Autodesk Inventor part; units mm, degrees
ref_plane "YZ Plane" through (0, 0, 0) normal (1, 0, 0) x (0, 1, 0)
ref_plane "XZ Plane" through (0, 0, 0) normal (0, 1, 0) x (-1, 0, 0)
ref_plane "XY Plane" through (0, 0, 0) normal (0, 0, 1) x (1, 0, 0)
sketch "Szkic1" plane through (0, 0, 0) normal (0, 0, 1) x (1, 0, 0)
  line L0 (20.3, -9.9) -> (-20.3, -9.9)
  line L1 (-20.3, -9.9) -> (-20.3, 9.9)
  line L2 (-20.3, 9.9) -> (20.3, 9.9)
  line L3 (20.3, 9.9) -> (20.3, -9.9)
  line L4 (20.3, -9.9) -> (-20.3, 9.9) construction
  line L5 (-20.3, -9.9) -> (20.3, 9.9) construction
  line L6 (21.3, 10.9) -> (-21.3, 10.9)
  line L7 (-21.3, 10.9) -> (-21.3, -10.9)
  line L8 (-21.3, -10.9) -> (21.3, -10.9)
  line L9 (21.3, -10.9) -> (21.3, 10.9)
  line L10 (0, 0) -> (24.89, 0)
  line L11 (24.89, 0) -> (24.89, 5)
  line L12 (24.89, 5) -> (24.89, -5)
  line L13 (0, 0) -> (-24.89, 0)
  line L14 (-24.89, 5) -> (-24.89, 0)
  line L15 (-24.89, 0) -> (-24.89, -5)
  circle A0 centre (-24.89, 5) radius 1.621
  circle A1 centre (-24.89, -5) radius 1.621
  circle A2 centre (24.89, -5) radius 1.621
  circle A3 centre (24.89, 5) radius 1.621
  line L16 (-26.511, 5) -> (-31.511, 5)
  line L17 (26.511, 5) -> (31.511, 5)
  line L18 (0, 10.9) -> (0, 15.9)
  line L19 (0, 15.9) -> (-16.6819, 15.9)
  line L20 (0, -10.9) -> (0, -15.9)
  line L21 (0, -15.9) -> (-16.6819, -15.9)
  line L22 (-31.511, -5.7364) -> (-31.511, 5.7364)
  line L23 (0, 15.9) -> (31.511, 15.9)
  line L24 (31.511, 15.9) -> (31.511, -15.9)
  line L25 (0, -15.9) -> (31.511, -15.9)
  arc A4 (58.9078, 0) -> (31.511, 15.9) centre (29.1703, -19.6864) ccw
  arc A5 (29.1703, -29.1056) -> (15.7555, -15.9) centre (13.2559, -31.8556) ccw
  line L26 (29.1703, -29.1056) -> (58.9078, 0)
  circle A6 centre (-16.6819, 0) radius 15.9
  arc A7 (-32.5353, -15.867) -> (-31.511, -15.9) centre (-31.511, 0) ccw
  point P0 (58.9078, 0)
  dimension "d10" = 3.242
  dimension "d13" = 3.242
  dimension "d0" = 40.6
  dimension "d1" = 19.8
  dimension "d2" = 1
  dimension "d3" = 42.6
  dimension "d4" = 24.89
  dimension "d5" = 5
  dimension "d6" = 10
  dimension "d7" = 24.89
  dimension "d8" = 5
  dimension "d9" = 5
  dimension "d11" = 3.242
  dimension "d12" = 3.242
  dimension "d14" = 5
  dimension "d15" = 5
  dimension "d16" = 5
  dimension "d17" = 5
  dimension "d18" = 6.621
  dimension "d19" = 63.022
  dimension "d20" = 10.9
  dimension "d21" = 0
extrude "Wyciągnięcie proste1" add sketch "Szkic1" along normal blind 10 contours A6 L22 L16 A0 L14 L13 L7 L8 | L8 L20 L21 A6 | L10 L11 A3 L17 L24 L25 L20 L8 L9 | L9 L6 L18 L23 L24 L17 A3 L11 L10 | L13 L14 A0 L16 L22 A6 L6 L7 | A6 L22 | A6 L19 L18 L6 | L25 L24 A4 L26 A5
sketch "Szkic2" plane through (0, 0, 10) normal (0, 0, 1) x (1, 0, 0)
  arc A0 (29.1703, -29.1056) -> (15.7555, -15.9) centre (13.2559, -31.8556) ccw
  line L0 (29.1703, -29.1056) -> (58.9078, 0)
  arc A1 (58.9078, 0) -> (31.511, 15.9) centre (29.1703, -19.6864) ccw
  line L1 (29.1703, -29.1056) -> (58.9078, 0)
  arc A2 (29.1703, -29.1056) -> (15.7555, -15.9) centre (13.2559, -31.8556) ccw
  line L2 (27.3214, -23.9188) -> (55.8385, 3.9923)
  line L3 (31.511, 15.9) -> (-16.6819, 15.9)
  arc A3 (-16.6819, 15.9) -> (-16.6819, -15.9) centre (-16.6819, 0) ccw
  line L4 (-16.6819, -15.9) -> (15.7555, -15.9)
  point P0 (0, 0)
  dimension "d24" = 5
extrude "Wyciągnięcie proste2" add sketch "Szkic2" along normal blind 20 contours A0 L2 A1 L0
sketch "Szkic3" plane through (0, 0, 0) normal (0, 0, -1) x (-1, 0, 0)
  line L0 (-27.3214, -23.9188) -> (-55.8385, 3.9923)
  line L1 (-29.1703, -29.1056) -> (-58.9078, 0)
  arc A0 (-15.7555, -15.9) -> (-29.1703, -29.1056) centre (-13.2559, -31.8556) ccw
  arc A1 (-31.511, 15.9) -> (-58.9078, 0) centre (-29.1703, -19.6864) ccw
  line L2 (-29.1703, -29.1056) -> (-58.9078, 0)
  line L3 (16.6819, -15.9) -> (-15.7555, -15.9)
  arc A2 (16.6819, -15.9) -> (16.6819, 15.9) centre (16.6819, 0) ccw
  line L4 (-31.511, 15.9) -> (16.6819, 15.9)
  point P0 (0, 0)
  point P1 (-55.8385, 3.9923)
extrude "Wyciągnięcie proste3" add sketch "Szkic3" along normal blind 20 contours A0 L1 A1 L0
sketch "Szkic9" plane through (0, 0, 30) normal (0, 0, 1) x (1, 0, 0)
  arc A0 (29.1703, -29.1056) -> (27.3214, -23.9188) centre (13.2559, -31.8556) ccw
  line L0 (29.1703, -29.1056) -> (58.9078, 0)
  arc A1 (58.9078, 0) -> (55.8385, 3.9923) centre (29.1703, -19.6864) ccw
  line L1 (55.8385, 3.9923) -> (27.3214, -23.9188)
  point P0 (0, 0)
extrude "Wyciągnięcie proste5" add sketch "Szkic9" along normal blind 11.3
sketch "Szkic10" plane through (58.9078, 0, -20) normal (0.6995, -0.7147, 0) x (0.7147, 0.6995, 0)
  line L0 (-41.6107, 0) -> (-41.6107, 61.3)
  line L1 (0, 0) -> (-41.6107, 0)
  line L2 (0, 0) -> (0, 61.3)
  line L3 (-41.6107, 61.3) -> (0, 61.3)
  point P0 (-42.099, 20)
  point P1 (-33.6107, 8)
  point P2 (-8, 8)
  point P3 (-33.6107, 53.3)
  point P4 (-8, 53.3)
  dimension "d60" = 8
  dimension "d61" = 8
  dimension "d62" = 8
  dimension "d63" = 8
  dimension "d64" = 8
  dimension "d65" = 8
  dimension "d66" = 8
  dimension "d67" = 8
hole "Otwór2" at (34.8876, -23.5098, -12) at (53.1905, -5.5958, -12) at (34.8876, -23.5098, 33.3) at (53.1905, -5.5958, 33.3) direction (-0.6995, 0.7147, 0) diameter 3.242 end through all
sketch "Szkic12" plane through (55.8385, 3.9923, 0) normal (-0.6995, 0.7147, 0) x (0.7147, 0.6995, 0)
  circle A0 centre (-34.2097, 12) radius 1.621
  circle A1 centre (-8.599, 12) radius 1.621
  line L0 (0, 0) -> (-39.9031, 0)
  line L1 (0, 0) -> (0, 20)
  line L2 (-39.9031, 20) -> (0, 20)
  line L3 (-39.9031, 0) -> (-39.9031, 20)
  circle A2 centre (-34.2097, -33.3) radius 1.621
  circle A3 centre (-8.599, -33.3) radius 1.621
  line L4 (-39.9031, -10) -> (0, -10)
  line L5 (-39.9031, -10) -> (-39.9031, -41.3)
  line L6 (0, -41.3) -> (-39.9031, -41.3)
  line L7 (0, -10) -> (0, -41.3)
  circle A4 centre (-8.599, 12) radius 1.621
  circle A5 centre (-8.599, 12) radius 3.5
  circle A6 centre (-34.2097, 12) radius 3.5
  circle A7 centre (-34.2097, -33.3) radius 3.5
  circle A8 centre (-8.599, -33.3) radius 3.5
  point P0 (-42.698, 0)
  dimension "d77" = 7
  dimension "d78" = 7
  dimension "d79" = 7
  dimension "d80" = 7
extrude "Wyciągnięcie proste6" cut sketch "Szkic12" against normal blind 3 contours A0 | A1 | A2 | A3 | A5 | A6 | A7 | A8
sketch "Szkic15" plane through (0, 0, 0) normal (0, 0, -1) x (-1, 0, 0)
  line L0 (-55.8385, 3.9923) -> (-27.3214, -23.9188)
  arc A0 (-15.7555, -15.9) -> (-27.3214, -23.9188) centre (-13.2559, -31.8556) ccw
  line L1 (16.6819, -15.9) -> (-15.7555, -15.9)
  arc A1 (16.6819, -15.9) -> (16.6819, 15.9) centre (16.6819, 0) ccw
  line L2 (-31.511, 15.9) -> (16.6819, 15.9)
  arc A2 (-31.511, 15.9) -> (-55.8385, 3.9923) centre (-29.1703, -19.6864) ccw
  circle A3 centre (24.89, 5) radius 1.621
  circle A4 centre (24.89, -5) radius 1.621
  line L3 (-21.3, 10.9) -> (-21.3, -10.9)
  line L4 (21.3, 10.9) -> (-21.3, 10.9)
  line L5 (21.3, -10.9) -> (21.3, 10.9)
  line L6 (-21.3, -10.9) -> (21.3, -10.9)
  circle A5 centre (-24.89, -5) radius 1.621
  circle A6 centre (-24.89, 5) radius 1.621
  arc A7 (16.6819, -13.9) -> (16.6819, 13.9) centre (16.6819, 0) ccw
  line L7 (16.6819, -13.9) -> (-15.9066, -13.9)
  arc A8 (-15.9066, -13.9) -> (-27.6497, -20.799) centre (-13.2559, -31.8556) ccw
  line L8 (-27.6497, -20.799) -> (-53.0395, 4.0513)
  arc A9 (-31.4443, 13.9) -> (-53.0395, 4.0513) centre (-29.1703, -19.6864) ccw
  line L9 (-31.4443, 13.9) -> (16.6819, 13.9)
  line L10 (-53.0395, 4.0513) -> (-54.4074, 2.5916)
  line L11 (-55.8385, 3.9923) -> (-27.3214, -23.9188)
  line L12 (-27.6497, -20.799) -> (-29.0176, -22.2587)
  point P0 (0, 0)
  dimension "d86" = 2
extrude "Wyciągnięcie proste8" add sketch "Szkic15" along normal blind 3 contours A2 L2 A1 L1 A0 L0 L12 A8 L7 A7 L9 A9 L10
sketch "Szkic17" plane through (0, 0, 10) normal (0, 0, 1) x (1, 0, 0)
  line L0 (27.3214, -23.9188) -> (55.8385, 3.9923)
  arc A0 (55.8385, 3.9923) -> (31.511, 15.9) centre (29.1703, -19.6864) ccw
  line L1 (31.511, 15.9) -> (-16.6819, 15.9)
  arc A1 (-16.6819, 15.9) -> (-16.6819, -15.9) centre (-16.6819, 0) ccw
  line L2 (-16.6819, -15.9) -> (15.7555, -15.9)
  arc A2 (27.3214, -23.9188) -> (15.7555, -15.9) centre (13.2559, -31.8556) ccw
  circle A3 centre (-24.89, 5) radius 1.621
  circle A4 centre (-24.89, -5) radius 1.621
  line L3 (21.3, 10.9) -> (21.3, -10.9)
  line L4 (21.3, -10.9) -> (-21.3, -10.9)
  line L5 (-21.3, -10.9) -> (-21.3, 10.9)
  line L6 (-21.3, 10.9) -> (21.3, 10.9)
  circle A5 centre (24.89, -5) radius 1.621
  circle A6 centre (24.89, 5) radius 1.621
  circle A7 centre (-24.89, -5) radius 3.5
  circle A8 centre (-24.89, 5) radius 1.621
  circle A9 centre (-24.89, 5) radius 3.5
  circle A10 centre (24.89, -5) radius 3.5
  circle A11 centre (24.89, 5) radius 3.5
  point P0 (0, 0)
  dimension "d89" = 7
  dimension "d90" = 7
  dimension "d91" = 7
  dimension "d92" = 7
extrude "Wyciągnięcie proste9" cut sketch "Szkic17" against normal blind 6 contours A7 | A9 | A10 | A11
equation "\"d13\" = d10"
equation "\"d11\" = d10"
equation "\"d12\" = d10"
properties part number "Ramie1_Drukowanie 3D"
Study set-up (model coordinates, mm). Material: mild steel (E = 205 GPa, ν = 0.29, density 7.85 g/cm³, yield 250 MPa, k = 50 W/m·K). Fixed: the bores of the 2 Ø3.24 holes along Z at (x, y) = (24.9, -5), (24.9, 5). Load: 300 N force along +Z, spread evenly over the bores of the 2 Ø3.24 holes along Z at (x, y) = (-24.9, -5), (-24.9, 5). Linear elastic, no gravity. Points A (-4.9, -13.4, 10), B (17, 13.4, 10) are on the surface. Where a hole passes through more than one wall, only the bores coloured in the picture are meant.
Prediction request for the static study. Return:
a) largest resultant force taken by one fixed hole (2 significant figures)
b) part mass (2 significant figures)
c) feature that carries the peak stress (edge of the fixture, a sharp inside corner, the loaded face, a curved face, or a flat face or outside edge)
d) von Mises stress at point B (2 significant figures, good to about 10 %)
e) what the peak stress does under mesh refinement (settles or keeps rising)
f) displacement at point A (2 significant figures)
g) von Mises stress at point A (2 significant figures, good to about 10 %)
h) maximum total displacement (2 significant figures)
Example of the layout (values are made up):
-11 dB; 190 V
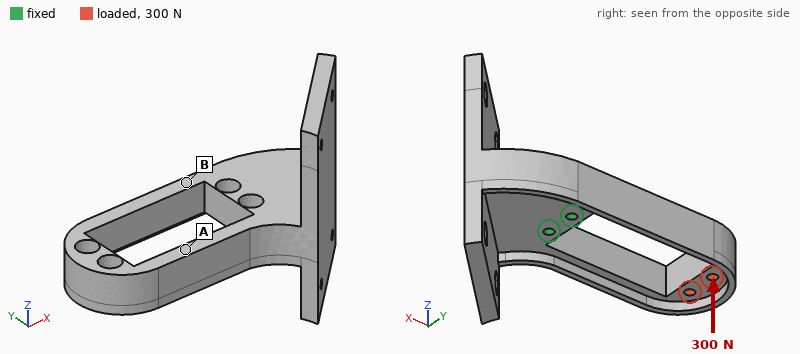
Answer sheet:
200 N; 210 g; edge of the fixture; 56 MPa; keeps rising; 0.063 mm; 27 MPa; 0.14 mm
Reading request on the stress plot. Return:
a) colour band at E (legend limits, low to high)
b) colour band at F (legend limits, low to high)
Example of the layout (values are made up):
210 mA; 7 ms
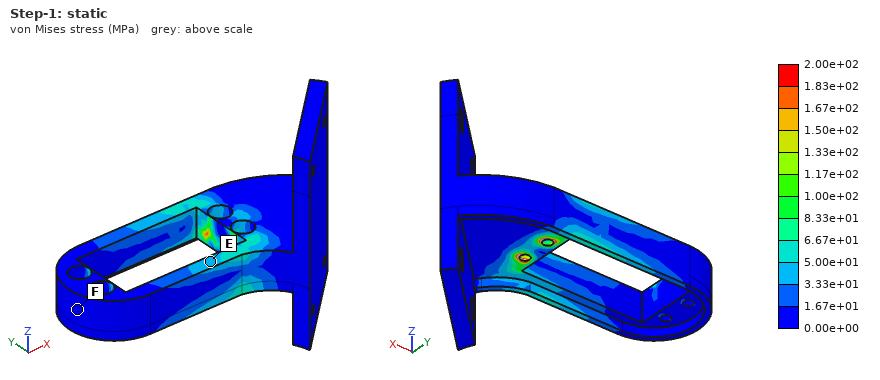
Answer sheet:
3.33e+01 to 5.00e+01 MPa; 0.00e+00 to 1.67e+01 MPa
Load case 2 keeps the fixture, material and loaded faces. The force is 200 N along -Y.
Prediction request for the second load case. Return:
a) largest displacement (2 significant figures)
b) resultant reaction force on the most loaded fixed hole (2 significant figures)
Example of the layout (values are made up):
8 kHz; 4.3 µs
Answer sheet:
58 µm; 750 N
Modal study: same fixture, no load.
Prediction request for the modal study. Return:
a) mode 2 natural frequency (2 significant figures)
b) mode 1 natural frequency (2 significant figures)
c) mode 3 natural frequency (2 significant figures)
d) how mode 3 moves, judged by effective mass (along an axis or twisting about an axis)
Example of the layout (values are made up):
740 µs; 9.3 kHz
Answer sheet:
1700 Hz; 1300 Hz; 2600 Hz; along Z
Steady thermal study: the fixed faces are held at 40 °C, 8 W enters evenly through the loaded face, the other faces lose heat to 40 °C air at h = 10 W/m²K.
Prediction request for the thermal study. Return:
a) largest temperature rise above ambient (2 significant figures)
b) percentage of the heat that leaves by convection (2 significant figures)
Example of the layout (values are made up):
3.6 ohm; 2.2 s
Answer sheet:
74 K; 30 %
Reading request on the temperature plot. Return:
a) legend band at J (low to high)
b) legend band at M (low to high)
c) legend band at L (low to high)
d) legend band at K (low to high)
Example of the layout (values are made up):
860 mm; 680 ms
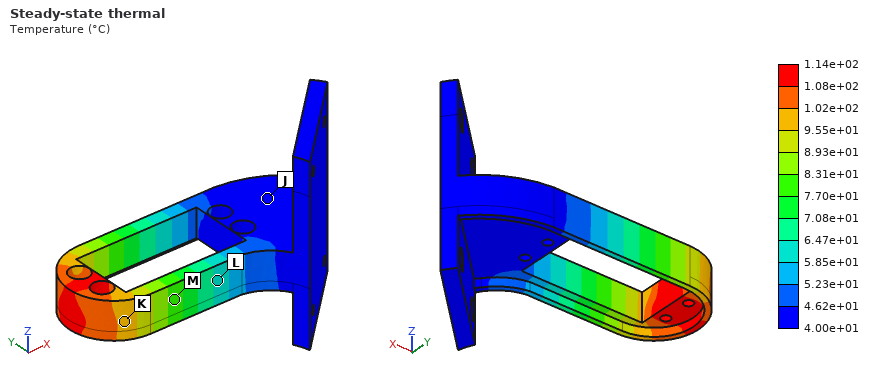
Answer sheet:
4.00e+01 to 4.62e+01 °C; 7.70e+01 to 8.31e+01 °C; 5.85e+01 to 6.47e+01 °C; 9.55e+01 to 1.02e+02 °C
